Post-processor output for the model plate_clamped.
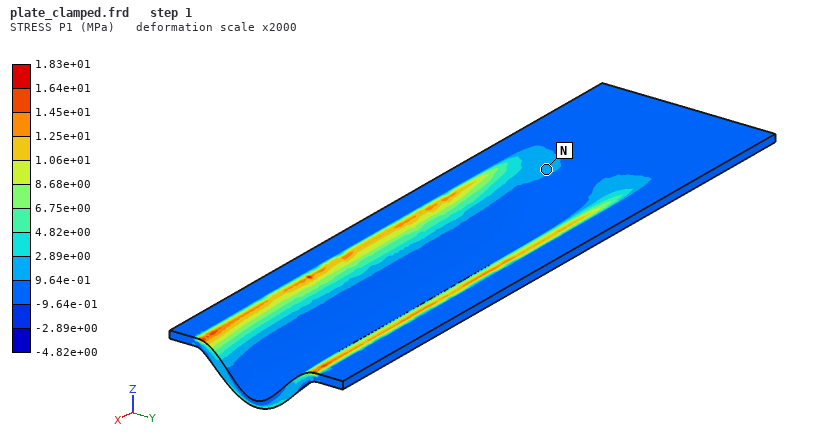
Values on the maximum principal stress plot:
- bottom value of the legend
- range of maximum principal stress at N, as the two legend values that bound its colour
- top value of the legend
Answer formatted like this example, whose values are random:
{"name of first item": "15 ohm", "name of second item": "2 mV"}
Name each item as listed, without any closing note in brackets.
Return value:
{"bottom value of the legend": "-4.82e+00 MPa", "range of maximum principal stress at N, as the two legend values that bound its colour": "9.64e-01 to 2.89e+00 MPa", "top value of the legend": "1.83e+01 MPa"}
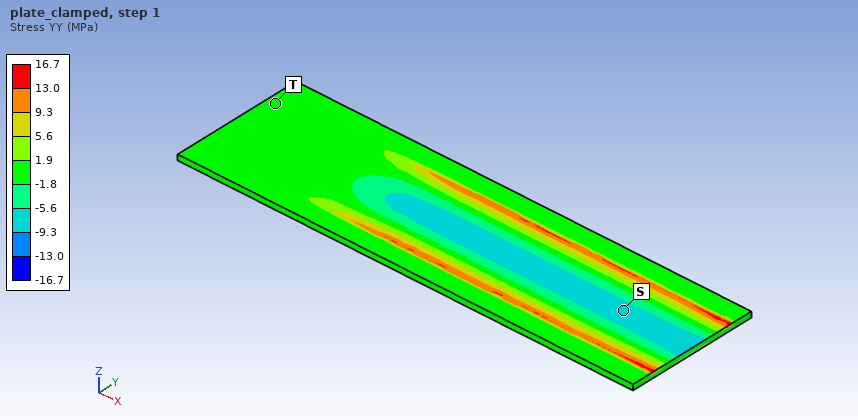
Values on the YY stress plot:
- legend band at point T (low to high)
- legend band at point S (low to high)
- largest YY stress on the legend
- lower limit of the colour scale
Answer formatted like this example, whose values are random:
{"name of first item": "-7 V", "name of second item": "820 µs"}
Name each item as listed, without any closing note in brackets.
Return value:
{"legend band at point T": "-1.8 to 1.9 MPa", "legend band at point S": "-9.3 to -5.6 MPa", "largest YY stress on the legend": "16.7 MPa", "lower limit of the colour scale": "-16.7 MPa"}
